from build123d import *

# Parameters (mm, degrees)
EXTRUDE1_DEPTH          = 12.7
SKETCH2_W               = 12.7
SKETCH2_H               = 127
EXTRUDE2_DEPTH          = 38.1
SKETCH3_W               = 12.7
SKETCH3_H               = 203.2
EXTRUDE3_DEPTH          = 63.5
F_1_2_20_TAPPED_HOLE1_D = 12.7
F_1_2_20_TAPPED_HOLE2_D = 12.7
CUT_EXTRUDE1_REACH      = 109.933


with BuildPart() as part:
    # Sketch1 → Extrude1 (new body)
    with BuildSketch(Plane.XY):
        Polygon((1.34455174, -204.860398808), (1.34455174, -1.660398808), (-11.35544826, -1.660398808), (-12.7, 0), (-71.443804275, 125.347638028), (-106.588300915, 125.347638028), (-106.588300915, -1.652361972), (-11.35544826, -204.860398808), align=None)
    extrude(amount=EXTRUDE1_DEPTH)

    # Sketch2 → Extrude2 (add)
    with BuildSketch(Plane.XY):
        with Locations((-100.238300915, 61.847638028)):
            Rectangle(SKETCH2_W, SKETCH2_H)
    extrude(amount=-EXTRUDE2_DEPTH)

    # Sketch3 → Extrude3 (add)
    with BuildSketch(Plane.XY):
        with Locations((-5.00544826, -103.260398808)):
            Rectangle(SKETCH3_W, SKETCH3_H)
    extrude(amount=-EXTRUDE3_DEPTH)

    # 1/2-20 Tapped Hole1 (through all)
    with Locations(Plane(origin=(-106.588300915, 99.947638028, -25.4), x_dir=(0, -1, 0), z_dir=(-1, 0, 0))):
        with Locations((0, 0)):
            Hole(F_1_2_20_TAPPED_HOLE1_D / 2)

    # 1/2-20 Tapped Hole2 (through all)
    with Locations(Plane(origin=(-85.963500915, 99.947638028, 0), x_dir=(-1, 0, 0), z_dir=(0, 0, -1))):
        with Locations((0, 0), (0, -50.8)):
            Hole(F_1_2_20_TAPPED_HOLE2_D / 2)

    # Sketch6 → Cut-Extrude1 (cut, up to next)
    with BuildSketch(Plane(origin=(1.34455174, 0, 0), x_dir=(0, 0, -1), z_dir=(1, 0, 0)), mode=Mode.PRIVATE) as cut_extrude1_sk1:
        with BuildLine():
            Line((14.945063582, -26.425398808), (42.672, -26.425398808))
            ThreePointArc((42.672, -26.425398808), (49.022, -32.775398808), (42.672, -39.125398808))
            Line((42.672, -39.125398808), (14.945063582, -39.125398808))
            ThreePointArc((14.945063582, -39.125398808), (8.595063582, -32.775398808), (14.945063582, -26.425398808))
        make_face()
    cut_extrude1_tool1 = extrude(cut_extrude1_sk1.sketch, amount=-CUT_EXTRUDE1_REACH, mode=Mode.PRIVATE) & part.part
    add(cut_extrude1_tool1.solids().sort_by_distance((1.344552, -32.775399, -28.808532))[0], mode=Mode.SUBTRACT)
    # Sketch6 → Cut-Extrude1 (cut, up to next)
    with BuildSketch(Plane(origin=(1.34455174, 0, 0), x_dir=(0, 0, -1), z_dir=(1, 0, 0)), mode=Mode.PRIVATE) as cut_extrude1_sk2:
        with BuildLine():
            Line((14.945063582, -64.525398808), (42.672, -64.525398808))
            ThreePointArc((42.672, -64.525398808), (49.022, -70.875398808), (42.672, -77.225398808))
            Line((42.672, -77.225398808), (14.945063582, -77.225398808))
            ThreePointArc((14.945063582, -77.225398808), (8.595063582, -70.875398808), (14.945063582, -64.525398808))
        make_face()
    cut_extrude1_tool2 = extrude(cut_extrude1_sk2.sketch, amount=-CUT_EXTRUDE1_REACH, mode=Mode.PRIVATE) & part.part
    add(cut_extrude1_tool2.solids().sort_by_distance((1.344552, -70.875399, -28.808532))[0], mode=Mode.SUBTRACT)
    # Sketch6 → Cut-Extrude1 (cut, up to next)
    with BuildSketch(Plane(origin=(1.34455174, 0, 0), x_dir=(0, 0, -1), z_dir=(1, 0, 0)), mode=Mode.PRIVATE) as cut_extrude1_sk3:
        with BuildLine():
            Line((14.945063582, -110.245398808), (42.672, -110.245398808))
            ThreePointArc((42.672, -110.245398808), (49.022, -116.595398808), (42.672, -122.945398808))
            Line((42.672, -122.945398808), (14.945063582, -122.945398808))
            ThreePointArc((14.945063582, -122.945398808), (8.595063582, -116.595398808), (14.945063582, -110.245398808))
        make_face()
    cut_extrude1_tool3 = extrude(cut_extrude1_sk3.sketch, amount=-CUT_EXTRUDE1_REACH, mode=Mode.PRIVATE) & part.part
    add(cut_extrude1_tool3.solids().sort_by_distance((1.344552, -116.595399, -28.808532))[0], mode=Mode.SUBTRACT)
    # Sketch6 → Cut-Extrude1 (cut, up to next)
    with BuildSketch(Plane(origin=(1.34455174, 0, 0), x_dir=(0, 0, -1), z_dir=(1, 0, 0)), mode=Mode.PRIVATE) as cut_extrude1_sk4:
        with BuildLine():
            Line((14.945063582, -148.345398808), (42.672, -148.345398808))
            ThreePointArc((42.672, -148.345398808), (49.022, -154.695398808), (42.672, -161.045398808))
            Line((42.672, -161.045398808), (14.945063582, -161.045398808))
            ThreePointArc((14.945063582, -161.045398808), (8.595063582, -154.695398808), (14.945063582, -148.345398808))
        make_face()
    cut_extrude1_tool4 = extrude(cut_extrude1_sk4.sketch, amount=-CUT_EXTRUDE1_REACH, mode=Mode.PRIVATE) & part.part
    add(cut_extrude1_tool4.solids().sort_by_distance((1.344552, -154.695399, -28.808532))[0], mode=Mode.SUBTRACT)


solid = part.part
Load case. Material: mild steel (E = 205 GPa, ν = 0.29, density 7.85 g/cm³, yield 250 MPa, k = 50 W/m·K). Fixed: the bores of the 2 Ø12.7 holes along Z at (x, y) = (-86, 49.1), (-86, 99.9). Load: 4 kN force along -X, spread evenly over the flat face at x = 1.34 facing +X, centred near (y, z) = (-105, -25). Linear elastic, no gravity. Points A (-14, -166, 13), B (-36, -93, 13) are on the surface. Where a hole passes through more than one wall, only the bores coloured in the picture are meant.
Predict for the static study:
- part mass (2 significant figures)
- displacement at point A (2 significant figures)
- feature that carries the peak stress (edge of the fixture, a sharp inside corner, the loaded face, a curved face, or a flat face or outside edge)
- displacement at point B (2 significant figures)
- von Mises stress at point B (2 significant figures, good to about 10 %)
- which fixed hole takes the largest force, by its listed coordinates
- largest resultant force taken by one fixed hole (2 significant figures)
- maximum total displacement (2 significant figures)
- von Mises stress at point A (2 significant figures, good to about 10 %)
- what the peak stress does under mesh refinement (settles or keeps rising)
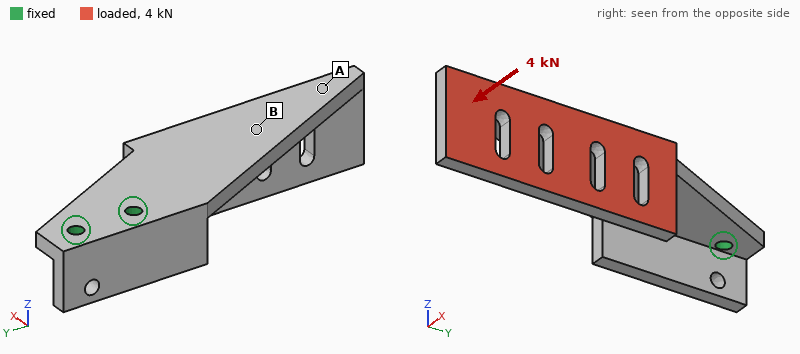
3.6 kg
0.33 mm
edge of the fixture
0.15 mm
28 MPa
(-86, 49.1)
14 kN
0.70 mm
14 MPa
keeps rising
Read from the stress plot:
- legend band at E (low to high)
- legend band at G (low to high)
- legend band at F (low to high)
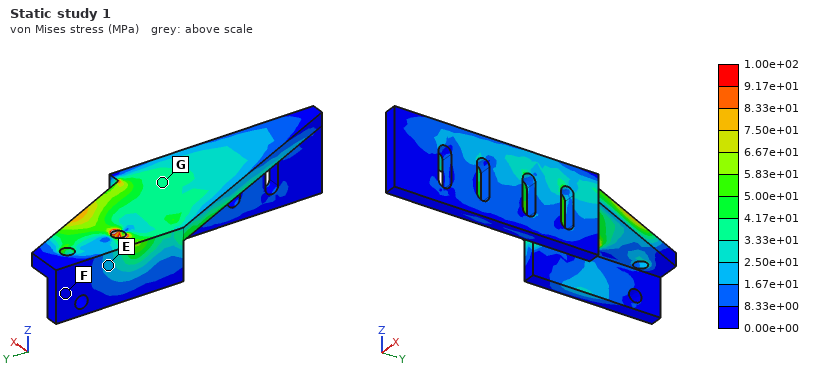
1.67e+01 to 2.50e+01 MPa
3.33e+01 to 4.17e+01 MPa
0.00e+00 to 8.33e+00 MPa
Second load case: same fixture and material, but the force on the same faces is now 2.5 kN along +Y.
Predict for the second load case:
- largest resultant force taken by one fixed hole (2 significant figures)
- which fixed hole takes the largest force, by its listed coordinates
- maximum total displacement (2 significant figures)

4.3 kN
(-86, 99.9)
0.48 mm
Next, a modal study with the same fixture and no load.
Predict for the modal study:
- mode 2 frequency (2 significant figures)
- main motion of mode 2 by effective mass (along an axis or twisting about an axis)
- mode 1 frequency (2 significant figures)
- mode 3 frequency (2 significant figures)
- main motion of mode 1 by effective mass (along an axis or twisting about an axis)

470 Hz
along X
160 Hz
810 Hz
along Z
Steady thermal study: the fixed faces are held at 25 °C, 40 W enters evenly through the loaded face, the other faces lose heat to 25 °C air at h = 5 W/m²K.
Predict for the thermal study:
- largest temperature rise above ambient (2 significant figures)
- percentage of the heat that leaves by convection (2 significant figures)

89 K
39 %
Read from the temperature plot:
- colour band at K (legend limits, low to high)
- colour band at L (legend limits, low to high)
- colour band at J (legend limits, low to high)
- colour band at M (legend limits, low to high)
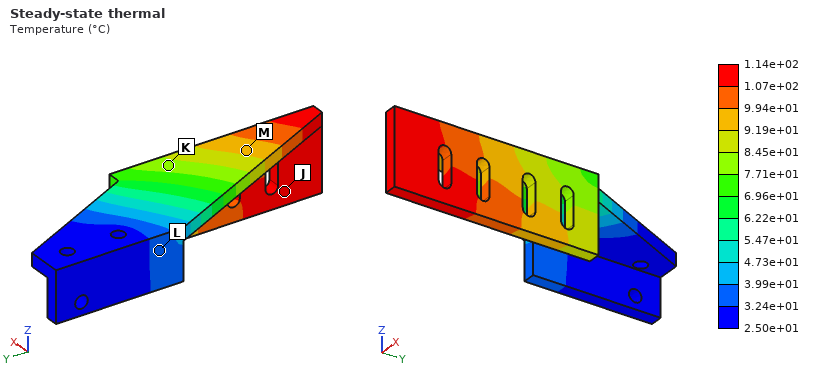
7.71e+01 to 8.45e+01 °C
3.24e+01 to 3.99e+01 °C
1.07e+02 to 1.14e+02 °C
9.19e+01 to 9.94e+01 °C
